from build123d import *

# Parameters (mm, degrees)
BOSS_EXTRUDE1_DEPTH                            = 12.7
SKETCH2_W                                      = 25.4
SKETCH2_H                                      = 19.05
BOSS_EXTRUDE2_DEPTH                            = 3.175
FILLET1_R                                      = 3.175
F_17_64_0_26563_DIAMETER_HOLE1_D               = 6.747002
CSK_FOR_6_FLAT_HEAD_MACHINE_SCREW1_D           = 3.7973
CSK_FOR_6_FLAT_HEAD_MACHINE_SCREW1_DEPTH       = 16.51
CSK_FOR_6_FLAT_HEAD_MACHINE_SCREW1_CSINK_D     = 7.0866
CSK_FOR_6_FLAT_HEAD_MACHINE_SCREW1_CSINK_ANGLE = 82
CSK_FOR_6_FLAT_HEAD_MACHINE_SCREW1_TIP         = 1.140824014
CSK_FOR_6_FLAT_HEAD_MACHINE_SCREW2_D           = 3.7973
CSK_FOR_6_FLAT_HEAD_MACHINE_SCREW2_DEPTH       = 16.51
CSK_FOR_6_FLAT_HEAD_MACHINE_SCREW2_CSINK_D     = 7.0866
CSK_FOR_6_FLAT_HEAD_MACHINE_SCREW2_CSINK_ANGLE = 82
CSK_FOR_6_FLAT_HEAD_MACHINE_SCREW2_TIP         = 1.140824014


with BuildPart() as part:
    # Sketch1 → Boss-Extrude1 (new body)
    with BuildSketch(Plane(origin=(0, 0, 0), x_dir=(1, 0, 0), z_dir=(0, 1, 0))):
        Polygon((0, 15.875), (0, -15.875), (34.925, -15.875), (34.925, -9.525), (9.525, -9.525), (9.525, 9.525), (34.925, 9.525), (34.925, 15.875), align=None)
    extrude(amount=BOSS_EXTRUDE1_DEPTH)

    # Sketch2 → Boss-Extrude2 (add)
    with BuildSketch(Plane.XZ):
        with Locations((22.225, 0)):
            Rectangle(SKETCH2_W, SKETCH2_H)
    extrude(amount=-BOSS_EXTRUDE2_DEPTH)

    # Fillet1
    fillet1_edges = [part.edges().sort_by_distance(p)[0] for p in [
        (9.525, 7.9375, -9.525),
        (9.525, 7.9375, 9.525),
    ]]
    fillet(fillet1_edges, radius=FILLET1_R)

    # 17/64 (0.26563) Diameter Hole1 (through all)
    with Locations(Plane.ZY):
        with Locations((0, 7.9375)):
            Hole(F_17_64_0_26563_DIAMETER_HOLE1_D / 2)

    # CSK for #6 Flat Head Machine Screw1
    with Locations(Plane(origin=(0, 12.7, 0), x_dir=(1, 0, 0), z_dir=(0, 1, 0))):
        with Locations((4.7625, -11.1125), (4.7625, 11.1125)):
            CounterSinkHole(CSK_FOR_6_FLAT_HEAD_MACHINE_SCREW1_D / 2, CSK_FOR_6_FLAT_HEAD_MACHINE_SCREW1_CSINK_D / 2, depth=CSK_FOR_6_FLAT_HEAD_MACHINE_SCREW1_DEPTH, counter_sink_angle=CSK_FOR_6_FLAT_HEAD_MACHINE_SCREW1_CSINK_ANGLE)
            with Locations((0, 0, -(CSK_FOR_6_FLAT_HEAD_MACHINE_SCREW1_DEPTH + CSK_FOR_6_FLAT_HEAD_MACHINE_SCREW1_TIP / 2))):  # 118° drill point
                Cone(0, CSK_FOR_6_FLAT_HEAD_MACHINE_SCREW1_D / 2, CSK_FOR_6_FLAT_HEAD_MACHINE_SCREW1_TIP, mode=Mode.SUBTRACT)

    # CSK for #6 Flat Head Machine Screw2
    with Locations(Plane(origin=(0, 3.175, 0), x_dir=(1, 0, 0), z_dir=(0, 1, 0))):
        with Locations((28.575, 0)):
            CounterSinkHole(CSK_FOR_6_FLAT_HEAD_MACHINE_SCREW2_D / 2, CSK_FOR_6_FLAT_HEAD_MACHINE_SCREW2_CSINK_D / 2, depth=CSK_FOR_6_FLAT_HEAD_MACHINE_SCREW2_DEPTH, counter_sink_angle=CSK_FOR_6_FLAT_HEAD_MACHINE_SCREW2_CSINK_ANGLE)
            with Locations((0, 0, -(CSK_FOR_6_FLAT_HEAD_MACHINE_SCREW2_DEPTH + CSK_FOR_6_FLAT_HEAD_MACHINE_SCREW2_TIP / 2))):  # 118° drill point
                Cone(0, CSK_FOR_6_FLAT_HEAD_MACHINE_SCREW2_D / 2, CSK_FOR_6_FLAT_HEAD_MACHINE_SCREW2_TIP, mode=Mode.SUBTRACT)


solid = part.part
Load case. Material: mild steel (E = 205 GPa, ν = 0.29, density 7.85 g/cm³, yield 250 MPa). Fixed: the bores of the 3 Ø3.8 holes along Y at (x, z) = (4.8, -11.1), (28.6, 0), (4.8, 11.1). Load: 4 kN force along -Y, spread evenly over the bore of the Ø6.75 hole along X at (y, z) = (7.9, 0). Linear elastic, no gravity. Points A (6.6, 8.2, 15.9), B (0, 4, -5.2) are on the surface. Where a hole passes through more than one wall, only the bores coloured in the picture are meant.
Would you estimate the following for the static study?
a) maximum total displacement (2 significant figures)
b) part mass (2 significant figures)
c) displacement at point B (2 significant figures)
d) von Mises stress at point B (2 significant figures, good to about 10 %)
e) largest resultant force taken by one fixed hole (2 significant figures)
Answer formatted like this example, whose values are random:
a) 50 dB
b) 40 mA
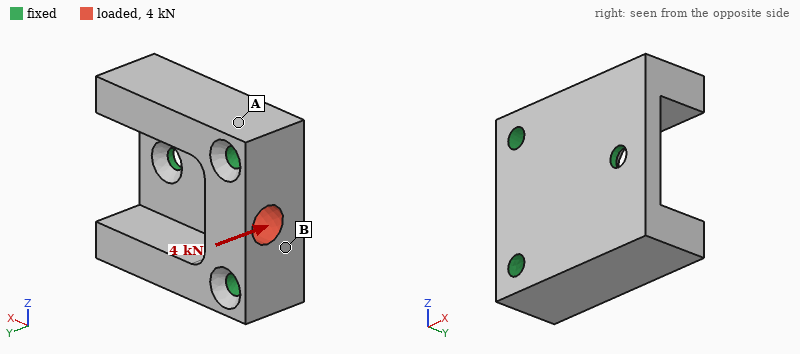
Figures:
a) 4.4 µm
b) 69 g
c) 1.6 µm
d) 34 MPa
e) 2.0 kN
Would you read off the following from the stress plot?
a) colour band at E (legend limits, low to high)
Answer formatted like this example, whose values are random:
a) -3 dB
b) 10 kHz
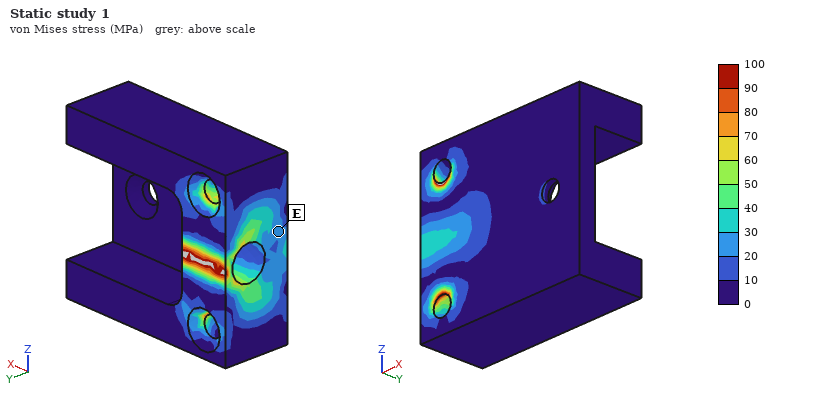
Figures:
a) 20 to 30 MPa
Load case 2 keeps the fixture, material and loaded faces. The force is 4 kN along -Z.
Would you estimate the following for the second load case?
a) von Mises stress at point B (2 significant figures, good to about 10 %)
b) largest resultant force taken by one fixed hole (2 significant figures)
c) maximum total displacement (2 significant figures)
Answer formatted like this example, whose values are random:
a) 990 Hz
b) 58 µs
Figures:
a) 14 MPa
b) 2.0 kN
c) 1.4 µm
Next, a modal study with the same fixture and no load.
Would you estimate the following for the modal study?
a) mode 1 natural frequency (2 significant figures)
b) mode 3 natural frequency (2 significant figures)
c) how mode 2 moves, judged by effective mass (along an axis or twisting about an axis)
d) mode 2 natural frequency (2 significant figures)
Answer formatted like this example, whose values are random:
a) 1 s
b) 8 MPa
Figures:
a) 13 kHz
b) 22 kHz
c) along Y
d) 14 kHz
